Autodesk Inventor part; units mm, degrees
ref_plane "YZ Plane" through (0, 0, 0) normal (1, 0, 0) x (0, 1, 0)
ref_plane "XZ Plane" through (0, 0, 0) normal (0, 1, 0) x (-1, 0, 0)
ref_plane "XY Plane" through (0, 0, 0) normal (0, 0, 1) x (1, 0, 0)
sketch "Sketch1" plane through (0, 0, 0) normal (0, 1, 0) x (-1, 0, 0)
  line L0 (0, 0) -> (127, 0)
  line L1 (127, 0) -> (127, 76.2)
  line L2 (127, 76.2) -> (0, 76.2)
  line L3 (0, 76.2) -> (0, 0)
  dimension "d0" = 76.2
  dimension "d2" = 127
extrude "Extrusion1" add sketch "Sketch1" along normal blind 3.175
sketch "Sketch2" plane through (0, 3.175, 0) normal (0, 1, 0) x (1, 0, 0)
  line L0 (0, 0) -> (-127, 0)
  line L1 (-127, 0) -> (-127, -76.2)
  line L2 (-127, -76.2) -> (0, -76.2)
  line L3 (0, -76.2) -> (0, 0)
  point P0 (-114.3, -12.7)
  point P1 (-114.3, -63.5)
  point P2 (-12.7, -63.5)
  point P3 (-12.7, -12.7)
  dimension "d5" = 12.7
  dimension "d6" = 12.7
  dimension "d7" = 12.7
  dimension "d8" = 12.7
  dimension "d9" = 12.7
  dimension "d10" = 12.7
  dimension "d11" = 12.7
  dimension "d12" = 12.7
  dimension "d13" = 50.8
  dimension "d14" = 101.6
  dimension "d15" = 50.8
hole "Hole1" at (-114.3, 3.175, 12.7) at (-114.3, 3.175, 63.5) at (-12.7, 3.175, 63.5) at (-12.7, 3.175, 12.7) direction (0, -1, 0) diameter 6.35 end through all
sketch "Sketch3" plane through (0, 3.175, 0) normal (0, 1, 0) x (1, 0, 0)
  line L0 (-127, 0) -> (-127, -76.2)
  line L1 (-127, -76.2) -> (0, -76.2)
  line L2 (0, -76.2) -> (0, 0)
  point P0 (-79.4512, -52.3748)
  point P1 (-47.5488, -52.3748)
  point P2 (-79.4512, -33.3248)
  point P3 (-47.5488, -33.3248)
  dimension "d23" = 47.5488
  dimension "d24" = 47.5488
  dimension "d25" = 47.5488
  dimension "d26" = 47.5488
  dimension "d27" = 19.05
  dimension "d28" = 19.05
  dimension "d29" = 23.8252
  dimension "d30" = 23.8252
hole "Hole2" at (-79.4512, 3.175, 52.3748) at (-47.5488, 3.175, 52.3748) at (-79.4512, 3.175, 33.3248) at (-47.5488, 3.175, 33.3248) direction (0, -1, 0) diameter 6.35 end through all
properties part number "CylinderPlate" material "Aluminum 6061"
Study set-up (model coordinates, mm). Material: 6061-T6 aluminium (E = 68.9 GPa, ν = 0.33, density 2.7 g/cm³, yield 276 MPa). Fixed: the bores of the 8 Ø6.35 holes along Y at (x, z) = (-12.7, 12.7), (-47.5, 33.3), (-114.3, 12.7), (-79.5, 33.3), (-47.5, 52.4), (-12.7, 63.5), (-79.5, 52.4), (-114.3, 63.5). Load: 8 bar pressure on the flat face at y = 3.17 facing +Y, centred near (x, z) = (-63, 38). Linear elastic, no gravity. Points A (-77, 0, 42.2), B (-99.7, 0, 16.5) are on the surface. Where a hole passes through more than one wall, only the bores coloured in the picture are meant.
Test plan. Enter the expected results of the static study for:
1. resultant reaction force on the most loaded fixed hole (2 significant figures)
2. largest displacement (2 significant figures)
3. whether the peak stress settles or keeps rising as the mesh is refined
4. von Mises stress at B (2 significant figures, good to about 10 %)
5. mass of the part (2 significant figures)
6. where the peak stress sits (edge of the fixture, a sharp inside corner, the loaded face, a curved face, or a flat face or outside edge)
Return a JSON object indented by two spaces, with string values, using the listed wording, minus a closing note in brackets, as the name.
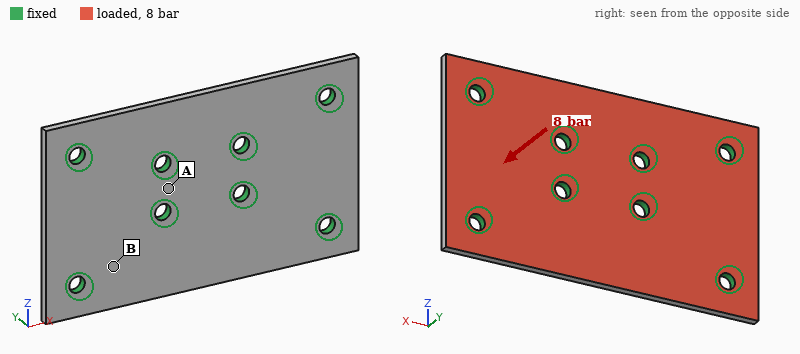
{
  "resultant reaction force on the most loaded fixed hole": "1.1 kN",
  "largest displacement": "0.36 mm",
  "whether the peak stress settles or keeps rising as the mesh is refined": "keeps rising",
  "von Mises stress at B": "67 MPa",
  "mass of the part": "81 g",
  "where the peak stress sits": "edge of the fixture"
}
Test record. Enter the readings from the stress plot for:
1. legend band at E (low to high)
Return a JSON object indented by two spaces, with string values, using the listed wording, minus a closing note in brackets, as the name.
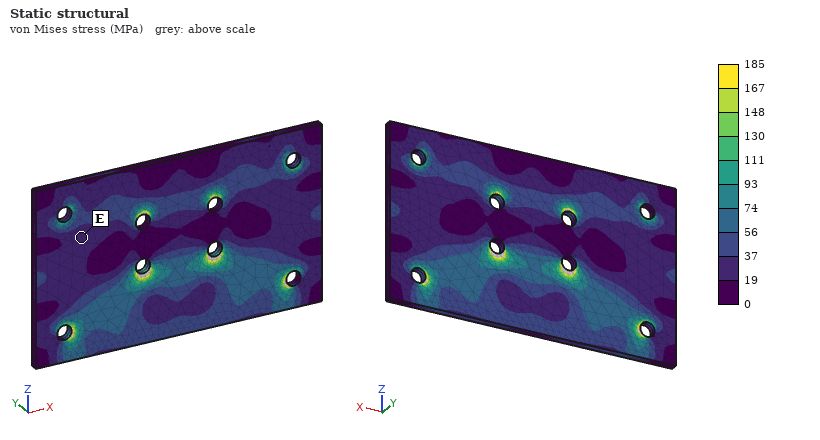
{
  "legend band at E": "19 to 37 MPa"
}
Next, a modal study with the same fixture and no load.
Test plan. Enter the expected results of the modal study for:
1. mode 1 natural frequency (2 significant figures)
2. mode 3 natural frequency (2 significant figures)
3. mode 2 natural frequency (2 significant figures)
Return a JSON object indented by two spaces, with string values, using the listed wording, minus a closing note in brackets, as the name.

{
  "mode 1 natural frequency": "3500 Hz",
  "mode 3 natural frequency": "6100 Hz",
  "mode 2 natural frequency": "5600 Hz"
}
